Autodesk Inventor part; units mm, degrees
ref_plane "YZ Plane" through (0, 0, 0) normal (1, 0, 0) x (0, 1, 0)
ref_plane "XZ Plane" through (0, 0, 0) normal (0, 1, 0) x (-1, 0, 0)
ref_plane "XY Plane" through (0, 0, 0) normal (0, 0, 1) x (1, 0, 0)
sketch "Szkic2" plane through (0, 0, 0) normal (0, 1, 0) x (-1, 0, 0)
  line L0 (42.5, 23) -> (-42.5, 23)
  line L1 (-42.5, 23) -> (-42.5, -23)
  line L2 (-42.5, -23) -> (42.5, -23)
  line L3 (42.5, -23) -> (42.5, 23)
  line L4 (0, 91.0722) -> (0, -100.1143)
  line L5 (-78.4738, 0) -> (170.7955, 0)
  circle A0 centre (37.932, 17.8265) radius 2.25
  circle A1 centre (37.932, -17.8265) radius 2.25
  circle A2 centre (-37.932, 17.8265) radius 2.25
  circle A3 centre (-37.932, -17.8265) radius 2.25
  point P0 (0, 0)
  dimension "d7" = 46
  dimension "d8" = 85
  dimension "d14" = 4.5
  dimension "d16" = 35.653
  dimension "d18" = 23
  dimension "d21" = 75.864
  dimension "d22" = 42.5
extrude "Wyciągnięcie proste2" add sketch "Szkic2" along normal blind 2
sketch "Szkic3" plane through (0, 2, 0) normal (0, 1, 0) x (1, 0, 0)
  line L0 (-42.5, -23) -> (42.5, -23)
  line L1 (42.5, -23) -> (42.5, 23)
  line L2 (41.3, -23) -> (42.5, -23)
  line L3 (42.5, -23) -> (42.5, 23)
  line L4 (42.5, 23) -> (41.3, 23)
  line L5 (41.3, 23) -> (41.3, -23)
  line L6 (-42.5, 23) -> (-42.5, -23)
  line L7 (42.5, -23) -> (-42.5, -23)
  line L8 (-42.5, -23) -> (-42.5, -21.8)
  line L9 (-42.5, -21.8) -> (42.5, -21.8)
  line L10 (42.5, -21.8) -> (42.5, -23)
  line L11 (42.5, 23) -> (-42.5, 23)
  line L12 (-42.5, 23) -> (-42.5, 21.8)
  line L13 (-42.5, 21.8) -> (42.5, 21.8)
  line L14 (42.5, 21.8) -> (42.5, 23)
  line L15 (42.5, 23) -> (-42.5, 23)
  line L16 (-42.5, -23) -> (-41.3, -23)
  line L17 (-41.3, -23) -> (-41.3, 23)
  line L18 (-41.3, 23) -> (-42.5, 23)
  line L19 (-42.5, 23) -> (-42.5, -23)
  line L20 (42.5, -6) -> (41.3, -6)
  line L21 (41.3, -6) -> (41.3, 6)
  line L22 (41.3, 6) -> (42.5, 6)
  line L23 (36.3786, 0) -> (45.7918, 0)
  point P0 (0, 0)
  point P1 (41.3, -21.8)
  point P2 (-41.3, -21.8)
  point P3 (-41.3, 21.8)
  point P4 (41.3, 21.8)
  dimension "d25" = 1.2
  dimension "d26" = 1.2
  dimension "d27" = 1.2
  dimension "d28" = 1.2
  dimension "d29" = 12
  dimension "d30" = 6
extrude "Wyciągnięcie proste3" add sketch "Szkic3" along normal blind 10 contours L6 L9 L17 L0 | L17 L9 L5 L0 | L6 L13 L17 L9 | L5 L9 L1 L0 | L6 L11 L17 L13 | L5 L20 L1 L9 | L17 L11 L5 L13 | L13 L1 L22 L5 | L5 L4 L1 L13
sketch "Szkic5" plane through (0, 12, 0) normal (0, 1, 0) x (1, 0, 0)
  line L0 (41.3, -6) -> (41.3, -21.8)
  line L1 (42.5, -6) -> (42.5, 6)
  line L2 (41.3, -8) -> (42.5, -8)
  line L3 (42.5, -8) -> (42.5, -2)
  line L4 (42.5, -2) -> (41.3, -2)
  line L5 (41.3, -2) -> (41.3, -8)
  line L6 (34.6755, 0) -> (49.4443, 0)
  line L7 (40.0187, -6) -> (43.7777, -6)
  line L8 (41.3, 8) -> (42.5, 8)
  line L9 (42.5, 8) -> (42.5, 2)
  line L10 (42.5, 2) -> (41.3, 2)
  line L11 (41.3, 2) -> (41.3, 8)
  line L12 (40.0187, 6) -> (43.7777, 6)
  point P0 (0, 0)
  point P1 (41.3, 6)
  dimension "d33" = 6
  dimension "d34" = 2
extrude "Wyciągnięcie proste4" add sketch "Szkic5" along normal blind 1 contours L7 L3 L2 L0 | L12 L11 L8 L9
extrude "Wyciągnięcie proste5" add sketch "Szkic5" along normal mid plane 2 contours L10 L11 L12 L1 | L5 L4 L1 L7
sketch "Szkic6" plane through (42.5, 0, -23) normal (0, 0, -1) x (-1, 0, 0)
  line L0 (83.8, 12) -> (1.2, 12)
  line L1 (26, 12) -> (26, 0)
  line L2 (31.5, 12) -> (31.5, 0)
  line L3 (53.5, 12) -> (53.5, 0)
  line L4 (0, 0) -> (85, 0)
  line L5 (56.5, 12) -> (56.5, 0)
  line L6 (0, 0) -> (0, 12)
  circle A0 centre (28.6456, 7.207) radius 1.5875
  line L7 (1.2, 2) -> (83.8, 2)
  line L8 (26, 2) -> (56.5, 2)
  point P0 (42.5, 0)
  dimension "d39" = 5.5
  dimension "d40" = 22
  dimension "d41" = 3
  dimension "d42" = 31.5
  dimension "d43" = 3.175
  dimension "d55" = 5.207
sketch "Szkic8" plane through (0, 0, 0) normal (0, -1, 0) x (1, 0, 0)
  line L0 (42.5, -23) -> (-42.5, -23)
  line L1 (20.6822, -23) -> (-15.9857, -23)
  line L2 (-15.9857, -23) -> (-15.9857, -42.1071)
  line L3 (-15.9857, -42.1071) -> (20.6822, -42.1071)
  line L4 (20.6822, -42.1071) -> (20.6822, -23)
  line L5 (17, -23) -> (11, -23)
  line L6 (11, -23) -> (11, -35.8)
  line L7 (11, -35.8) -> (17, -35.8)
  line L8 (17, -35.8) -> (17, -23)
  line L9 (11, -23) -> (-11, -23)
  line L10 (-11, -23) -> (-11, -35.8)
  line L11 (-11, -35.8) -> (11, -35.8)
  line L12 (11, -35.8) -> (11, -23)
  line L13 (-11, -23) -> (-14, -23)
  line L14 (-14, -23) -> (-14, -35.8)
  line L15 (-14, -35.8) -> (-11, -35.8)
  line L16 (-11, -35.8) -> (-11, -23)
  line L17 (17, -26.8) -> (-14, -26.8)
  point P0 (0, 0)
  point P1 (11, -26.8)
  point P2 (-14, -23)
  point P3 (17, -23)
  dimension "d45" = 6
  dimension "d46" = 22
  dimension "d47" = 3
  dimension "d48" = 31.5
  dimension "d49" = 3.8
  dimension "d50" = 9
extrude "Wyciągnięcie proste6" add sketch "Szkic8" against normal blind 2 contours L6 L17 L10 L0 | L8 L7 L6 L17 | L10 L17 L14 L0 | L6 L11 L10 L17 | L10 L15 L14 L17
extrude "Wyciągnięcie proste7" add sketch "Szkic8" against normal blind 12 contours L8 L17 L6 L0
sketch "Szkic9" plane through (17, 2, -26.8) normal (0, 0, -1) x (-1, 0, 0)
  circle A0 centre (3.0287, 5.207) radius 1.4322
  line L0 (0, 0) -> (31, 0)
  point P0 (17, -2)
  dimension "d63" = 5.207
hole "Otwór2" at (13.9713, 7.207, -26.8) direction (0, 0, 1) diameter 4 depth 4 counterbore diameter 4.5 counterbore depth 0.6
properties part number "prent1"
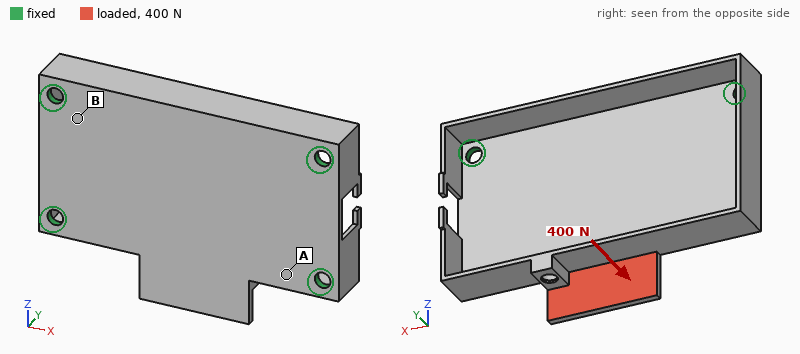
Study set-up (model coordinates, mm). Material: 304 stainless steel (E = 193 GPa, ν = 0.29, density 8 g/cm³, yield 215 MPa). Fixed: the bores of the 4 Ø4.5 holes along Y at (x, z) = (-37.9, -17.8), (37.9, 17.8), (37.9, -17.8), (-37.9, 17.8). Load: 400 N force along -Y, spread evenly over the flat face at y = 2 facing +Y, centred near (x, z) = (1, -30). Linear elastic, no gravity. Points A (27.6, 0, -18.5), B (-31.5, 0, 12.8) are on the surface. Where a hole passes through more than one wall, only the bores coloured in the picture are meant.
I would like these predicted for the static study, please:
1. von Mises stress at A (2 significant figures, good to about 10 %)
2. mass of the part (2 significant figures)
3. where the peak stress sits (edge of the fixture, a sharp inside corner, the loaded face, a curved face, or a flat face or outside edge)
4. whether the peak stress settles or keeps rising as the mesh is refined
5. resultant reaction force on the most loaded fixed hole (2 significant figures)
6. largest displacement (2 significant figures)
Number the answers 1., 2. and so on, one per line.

1. 59 MPa
2. 93 g
3. edge of the fixture
4. keeps rising
5. 410 N
6. 0.15 mm
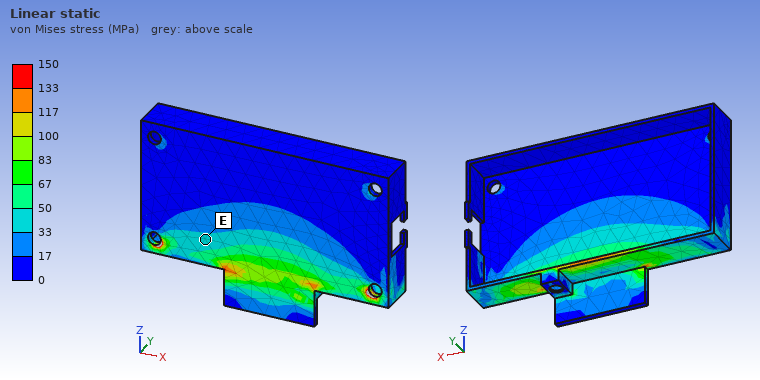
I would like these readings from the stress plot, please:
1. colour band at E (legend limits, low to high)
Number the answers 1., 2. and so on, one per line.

1. 33 to 50 MPa
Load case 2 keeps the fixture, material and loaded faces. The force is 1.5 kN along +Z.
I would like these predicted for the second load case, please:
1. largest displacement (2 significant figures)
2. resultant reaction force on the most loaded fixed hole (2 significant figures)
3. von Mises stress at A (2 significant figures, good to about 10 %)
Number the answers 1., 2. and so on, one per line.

1. 62 µm
2. 520 N
3. 14 MPa
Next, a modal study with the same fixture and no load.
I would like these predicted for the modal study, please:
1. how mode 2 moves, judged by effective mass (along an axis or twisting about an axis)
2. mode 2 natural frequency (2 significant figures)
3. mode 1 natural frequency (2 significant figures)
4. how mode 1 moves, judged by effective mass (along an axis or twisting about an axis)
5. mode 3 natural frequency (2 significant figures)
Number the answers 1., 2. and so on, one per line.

1. along Y
2. 3500 Hz
3. 2900 Hz
4. along Y
5. 5700 Hz
